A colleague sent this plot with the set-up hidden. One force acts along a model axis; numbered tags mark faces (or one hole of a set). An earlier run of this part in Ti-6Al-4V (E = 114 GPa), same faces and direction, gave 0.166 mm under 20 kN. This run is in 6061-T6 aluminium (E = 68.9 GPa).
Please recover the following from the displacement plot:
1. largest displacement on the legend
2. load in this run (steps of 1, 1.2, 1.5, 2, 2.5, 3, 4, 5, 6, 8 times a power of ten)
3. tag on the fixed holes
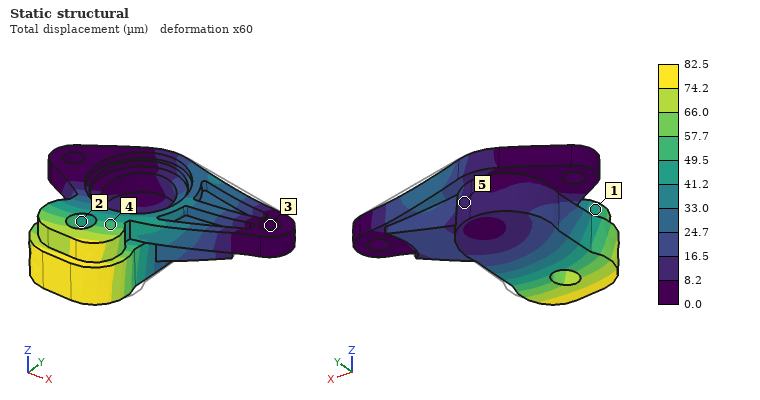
82.5 µm
6 kN
3
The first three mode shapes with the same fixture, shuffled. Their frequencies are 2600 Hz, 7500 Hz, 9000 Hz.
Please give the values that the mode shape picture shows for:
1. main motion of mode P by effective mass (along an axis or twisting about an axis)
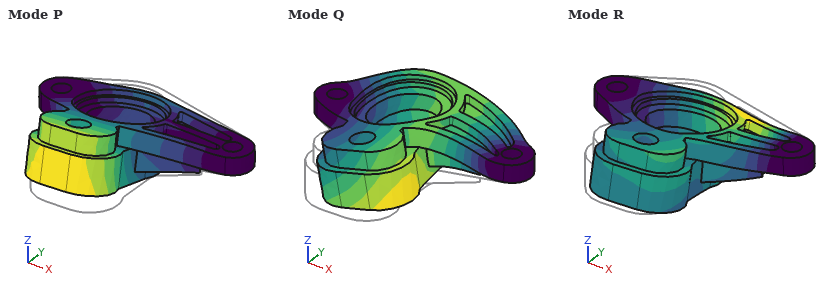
along Z
